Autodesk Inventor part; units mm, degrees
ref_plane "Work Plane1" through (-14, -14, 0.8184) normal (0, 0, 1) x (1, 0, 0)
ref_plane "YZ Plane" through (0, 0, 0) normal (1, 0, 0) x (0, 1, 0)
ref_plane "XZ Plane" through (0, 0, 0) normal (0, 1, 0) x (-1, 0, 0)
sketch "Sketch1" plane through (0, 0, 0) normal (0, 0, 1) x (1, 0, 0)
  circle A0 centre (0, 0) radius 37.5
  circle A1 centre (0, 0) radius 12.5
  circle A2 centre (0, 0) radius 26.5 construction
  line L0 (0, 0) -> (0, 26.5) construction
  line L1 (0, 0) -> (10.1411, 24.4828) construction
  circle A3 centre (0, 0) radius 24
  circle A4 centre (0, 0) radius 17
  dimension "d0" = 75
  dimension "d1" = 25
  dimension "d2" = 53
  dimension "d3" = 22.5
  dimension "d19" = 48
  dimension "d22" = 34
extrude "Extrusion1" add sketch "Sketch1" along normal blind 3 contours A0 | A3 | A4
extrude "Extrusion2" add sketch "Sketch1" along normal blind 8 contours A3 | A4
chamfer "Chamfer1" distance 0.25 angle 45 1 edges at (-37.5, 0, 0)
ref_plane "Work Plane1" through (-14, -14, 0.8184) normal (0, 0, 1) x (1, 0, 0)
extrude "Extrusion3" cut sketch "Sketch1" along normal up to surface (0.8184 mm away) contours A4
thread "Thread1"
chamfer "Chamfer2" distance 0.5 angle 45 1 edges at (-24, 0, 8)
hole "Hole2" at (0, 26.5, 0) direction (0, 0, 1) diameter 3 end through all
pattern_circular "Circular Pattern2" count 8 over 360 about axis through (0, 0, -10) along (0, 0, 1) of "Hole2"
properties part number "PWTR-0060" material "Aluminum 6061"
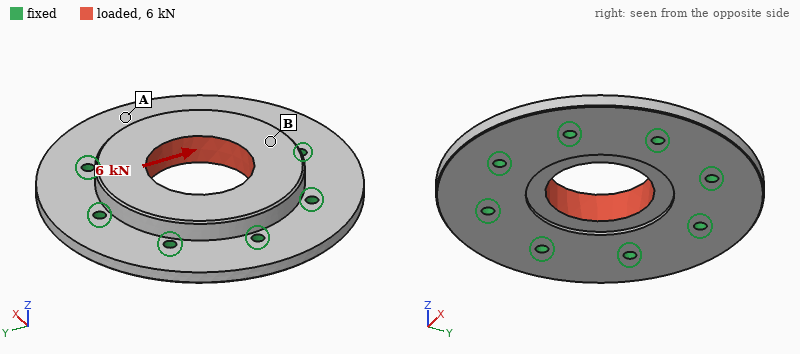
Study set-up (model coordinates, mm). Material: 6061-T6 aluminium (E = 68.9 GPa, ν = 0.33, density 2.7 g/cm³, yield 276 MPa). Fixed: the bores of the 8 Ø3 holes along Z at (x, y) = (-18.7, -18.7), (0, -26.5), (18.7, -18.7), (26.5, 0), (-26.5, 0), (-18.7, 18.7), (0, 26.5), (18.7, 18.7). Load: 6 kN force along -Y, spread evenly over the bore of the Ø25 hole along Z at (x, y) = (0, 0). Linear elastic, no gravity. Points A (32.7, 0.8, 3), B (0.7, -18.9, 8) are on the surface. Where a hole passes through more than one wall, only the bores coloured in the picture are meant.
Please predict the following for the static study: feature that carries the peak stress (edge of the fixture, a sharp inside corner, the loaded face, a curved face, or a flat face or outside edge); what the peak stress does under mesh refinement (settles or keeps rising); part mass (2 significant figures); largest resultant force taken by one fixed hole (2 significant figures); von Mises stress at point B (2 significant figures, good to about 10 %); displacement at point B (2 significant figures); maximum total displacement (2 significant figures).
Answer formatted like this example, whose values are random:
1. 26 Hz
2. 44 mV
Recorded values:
1. edge of the fixture
2. keeps rising
3. 48 g
4. 1.0 kN
5. 14 MPa
6. 6.1 µm
7. 8.4 µm
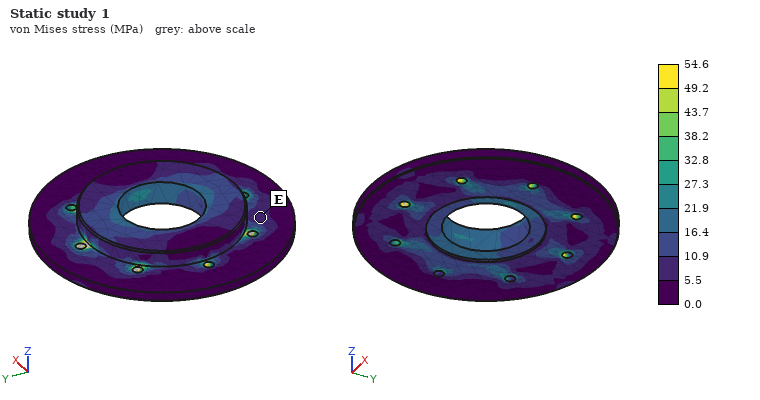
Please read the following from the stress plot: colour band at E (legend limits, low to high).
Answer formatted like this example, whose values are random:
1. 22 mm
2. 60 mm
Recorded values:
1. 5.5 to 10.9 MPa
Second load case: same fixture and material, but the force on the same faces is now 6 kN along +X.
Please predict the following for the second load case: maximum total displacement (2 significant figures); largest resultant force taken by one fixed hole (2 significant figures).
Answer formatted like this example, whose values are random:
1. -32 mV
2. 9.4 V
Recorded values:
1. 8.4 µm
2. 1.0 kN
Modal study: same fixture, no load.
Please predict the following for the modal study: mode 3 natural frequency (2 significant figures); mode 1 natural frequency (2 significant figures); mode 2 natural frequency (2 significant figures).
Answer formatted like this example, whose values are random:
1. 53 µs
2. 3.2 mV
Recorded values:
1. 16 kHz
2. 16 kHz
3. 16 kHz
